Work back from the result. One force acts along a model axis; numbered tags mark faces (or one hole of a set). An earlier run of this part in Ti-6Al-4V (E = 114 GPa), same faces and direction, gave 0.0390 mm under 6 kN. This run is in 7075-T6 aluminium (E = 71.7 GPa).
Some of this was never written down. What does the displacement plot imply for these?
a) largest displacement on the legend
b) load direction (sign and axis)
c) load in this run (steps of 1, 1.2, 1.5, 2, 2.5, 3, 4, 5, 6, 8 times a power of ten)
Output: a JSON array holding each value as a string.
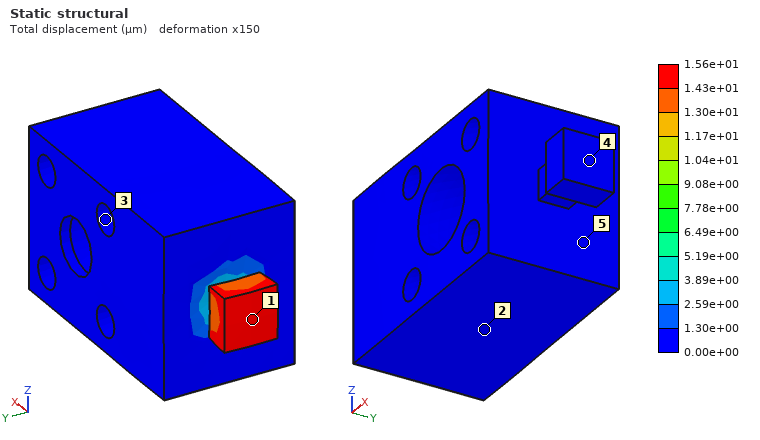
["1.56e+01 µm", "+X", "1.5 kN"]
